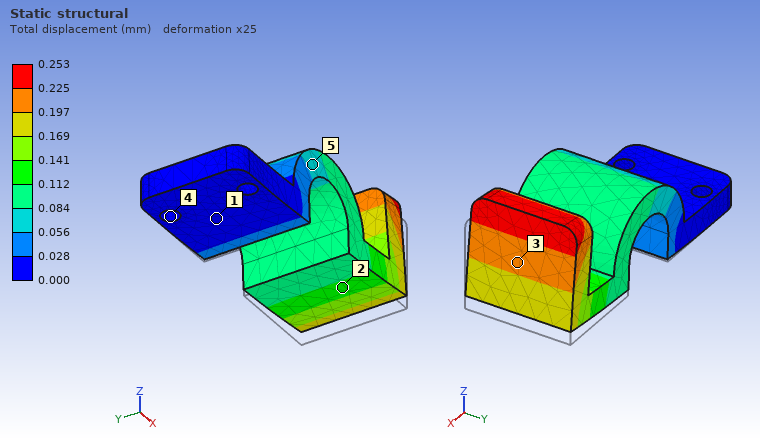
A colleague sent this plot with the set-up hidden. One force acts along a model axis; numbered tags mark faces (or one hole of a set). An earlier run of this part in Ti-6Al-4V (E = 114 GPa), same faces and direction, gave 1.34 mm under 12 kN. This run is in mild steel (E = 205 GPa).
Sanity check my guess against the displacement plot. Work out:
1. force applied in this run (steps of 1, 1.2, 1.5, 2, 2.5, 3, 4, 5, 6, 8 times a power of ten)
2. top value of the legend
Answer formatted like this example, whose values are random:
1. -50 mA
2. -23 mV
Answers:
1. 4 kN
2. 0.253 mm
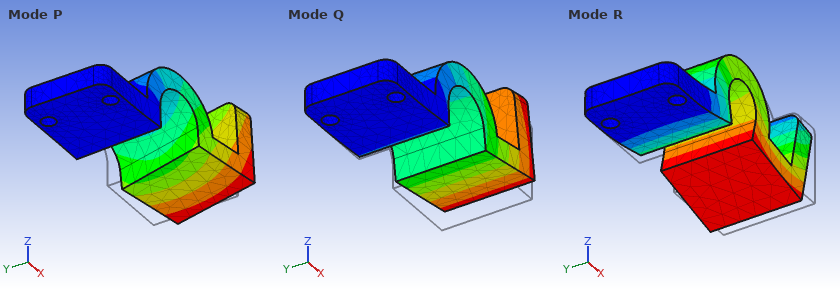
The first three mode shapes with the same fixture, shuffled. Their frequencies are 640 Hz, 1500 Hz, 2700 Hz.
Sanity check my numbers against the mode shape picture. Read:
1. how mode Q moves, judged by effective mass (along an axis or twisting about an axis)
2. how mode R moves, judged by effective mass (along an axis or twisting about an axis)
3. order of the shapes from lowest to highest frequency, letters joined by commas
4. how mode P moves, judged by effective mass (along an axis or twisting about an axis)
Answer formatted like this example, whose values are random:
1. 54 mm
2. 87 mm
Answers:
1. along Z
2. along X
3. Q, P, R
4. along Y
